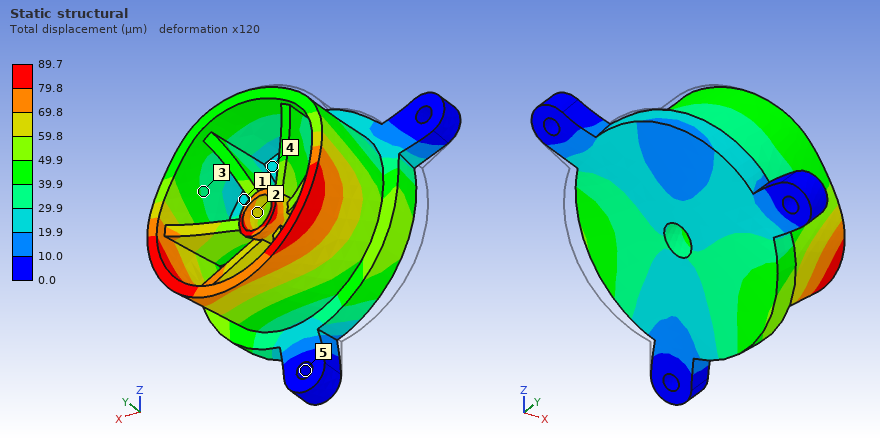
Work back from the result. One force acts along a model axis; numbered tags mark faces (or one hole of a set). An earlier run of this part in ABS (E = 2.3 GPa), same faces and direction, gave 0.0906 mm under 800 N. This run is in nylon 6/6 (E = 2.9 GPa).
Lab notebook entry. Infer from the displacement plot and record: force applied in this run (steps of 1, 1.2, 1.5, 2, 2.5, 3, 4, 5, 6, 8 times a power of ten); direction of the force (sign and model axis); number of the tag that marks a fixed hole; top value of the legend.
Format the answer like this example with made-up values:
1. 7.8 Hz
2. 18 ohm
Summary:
1. 1 kN
2. +X
3. 5
4. 89.7 µm
